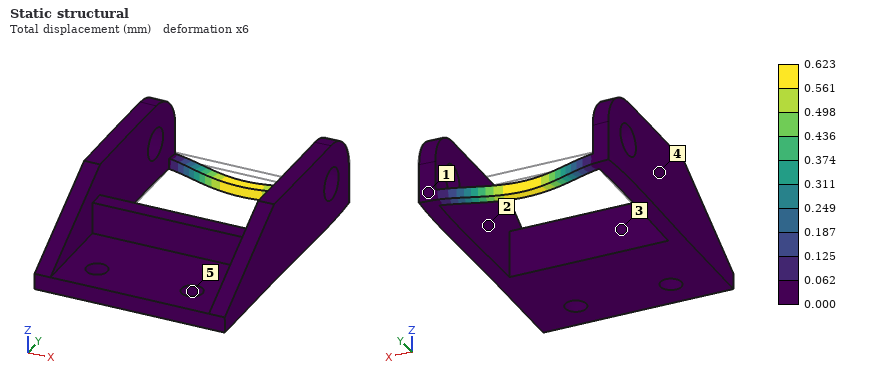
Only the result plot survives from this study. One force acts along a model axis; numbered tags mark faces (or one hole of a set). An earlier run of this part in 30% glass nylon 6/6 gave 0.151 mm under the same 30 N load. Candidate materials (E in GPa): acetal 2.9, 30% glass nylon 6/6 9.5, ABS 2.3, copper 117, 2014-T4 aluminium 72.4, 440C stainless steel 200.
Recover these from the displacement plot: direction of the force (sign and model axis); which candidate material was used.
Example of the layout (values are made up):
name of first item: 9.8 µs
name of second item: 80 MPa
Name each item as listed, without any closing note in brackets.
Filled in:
direction of the force: -Y
which candidate material was used: ABS
